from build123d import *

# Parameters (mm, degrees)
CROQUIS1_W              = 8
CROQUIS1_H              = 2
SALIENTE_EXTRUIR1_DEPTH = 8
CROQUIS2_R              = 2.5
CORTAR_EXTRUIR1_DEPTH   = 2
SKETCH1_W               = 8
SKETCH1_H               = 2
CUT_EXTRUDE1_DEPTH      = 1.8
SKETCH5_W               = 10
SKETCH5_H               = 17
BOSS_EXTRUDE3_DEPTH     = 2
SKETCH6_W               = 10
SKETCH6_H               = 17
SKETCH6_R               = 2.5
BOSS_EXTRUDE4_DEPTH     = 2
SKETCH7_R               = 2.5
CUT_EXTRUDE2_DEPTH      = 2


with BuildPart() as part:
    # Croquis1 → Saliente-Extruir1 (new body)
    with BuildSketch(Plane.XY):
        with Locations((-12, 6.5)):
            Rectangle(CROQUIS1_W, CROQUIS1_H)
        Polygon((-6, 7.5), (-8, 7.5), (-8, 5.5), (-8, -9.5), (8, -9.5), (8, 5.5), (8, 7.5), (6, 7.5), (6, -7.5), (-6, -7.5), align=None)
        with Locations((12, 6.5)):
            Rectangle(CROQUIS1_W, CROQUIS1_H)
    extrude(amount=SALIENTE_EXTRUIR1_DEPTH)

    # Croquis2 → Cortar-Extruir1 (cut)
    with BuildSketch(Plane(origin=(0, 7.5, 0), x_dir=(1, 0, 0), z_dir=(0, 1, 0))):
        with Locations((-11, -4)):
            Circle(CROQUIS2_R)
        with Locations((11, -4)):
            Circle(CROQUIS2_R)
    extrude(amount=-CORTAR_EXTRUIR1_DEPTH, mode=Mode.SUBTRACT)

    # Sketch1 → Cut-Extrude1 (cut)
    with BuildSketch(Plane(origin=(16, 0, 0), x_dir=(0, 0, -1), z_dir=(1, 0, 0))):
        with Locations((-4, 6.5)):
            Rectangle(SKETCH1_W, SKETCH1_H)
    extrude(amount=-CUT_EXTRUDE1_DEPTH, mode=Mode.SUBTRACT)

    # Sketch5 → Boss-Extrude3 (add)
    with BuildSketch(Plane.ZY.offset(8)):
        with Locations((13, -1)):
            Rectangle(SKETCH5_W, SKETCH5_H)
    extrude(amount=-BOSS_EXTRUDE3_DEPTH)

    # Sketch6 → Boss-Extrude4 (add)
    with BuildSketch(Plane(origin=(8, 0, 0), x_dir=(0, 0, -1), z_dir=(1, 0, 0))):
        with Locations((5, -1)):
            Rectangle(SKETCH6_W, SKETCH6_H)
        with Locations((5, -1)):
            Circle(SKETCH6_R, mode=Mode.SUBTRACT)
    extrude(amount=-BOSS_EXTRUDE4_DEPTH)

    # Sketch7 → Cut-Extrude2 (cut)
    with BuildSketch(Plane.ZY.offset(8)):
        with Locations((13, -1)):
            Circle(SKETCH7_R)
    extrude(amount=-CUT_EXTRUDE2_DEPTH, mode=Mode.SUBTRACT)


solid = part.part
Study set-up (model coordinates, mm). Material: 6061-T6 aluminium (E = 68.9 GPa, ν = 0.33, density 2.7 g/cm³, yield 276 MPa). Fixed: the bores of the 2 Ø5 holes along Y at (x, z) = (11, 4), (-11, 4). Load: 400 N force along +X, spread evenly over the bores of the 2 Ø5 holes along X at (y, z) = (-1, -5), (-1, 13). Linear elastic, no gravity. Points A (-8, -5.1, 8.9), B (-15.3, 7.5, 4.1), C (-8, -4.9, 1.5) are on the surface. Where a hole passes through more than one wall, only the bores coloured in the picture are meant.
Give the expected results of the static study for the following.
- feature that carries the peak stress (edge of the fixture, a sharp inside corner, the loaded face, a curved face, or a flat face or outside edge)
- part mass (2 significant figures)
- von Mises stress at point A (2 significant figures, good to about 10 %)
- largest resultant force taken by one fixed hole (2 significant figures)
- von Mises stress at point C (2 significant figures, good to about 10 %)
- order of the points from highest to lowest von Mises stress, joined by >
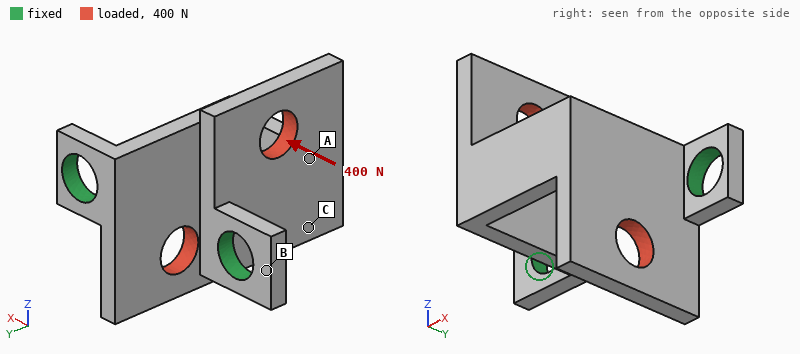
a flat face or outside edge
4.0 g
93 MPa
210 N
60 MPa
A > C > B
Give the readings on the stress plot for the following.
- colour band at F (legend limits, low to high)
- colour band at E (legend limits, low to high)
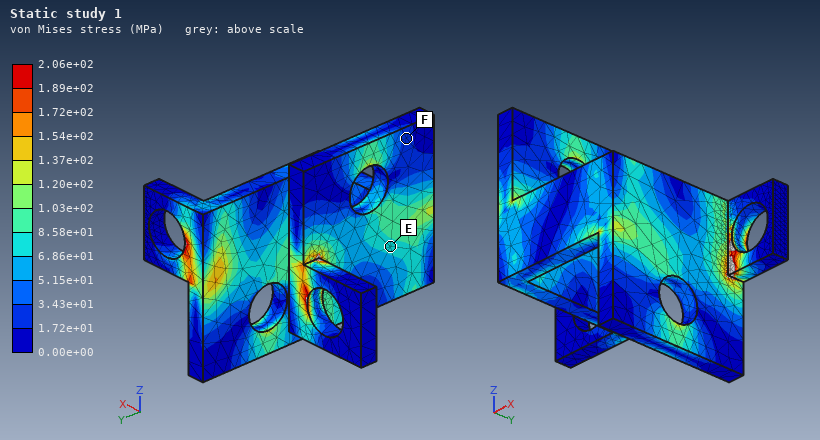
1.72e+01 to 3.43e+01 MPa
6.86e+01 to 8.58e+01 MPa
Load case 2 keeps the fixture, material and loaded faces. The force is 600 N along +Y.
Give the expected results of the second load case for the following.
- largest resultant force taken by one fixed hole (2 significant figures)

300 N
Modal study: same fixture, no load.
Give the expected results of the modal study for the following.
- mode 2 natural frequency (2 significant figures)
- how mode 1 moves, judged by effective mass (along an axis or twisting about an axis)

6300 Hz
along X
